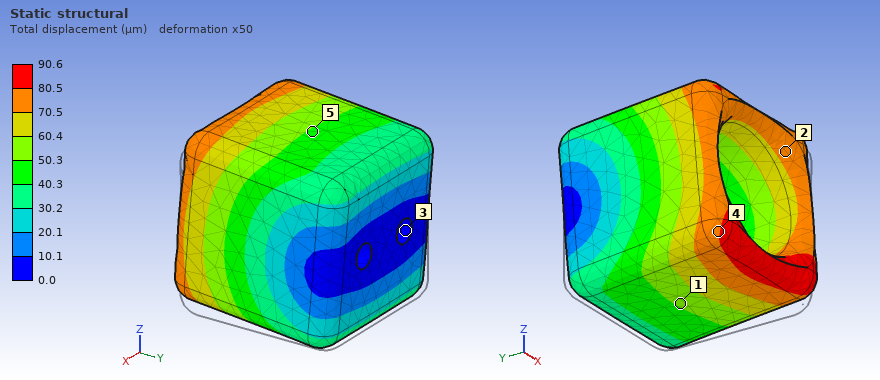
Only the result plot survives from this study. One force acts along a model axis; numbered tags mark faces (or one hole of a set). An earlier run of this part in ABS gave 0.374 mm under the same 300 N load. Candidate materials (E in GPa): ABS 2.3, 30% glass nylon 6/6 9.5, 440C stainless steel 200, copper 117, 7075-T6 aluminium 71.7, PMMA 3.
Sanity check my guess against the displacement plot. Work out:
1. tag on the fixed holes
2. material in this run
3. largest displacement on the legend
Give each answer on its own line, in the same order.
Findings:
3
30% glass nylon 6/6
90.6 µm
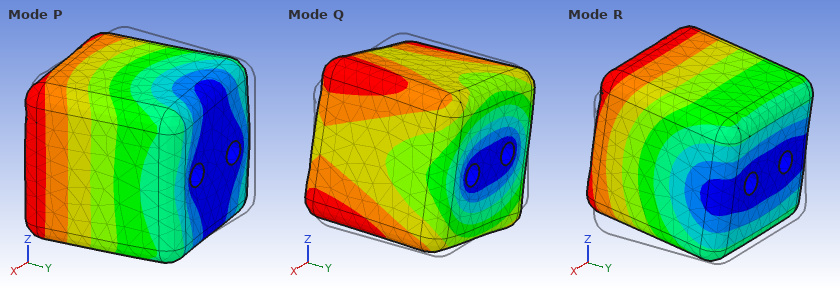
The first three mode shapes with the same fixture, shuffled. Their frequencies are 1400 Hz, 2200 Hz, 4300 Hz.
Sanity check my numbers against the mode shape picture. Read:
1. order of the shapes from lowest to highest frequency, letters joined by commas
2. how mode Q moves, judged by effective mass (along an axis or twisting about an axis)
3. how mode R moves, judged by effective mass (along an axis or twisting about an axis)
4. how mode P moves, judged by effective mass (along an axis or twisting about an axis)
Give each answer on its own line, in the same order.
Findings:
R, P, Q
twisting about Y
along Z
along X
